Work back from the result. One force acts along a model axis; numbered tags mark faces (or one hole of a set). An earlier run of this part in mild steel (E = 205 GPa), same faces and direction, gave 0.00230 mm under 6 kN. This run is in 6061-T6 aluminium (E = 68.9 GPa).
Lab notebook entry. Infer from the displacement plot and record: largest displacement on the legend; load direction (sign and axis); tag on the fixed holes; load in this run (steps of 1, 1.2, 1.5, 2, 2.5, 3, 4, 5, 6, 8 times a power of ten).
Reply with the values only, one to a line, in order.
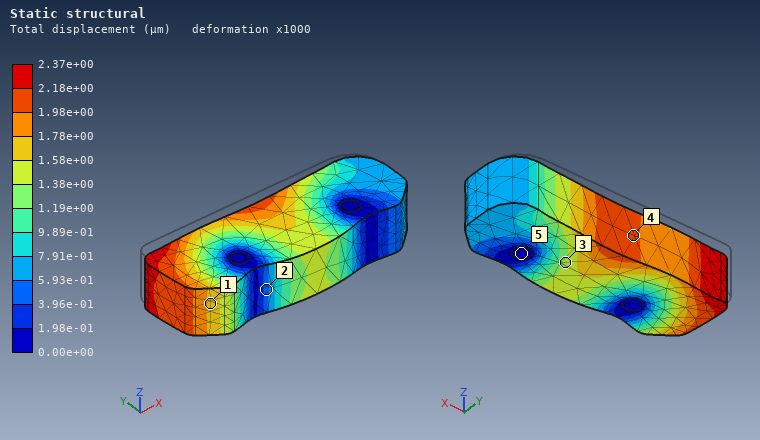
2.37e+00 µm
-Y
5
2 kN
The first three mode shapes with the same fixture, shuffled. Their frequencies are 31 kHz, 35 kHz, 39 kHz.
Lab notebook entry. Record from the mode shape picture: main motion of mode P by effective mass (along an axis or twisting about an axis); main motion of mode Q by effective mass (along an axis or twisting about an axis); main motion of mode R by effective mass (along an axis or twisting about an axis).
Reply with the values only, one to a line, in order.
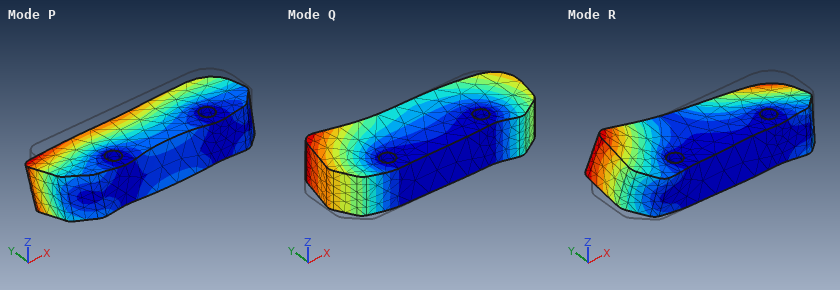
along Z
along X
twisting about Y
